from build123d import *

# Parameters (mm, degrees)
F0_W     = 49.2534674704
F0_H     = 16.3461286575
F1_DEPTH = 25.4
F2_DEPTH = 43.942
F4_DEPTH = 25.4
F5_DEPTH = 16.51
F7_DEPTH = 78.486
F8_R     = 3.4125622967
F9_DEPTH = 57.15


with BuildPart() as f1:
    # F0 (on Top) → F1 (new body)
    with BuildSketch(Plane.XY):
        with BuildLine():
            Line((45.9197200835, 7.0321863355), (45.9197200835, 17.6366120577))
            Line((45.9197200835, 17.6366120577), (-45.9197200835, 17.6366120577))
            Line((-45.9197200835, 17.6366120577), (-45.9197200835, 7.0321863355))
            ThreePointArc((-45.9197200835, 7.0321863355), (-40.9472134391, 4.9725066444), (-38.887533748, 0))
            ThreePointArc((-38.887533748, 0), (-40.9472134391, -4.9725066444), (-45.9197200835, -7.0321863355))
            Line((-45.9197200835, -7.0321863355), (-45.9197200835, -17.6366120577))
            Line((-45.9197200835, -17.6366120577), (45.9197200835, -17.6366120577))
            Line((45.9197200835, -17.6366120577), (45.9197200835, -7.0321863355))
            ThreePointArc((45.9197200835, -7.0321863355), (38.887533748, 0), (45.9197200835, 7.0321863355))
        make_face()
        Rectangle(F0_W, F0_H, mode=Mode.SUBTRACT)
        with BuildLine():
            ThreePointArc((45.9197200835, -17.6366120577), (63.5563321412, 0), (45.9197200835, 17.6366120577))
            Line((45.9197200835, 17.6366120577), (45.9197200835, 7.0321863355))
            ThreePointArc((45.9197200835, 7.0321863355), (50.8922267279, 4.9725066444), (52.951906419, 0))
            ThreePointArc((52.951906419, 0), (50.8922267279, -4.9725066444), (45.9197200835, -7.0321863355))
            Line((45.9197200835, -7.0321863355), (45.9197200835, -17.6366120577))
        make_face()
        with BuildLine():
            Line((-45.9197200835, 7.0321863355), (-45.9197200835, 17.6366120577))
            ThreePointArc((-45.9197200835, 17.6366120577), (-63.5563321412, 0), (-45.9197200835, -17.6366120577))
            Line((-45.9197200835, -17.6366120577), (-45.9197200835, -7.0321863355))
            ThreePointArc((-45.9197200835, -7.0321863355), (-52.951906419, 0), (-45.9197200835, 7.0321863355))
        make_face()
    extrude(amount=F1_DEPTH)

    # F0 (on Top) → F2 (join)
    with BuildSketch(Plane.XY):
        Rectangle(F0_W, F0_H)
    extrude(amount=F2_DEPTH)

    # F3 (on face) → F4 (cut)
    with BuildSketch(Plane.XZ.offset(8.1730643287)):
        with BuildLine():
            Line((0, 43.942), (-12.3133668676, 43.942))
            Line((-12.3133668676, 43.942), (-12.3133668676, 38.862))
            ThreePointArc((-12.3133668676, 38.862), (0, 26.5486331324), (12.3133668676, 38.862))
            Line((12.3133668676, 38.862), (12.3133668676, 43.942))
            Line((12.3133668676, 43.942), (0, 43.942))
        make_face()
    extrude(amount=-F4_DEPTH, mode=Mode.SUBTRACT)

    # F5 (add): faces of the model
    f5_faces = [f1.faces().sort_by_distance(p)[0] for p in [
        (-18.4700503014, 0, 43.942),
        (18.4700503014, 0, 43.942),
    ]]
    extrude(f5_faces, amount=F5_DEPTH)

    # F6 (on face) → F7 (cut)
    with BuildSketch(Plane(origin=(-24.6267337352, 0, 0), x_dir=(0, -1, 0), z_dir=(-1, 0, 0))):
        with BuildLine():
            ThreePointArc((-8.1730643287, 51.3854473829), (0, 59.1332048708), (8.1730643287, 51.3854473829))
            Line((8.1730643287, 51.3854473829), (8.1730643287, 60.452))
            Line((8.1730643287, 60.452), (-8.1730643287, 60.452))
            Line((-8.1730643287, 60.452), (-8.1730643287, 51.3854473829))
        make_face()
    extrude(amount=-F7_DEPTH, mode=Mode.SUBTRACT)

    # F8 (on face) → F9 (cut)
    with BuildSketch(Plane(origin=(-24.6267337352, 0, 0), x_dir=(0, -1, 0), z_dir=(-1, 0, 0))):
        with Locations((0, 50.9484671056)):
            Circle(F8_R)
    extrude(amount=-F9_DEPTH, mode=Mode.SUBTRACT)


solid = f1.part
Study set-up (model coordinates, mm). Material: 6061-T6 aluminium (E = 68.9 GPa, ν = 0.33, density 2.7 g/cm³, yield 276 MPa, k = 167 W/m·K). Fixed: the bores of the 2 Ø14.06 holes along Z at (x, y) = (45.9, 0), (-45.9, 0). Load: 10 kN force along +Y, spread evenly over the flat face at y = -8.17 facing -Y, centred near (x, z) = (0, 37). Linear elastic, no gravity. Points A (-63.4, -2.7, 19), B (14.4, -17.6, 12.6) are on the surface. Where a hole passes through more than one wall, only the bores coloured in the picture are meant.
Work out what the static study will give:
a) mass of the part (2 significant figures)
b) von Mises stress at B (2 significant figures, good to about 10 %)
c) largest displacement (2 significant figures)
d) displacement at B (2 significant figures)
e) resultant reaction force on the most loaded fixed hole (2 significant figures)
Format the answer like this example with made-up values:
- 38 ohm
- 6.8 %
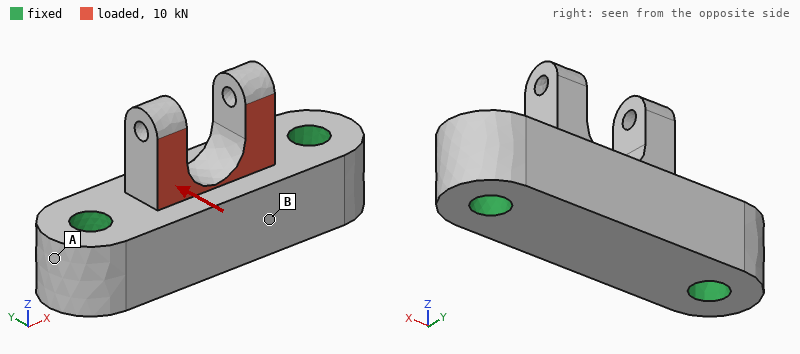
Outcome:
- 300 g
- 20 MPa
- 0.13 mm
- 0.021 mm
- 5.0 kN
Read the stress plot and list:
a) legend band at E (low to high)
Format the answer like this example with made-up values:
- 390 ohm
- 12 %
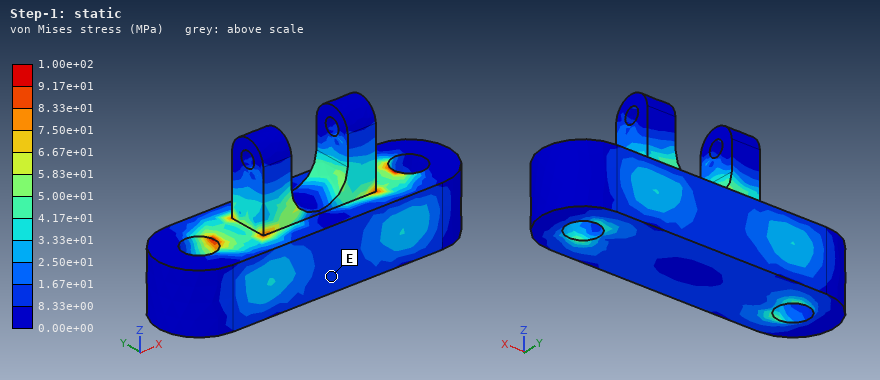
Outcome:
- 8.33e+00 to 1.67e+01 MPa
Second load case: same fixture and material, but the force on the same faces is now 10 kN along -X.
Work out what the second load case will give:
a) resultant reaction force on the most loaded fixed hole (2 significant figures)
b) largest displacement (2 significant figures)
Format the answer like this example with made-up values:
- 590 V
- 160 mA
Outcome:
- 6.0 kN
- 88 µm
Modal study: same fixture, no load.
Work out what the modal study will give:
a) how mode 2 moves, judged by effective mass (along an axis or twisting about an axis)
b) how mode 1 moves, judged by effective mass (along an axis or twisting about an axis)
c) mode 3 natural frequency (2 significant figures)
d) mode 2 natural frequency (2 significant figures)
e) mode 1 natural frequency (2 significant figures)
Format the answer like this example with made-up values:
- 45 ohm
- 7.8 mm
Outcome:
- along Z
- along Y
- 10 kHz
- 9500 Hz
- 7900 Hz
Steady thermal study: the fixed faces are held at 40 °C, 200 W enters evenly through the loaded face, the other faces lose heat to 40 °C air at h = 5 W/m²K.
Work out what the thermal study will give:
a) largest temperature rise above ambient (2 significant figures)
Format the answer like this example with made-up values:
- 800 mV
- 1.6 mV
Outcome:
- 63 K
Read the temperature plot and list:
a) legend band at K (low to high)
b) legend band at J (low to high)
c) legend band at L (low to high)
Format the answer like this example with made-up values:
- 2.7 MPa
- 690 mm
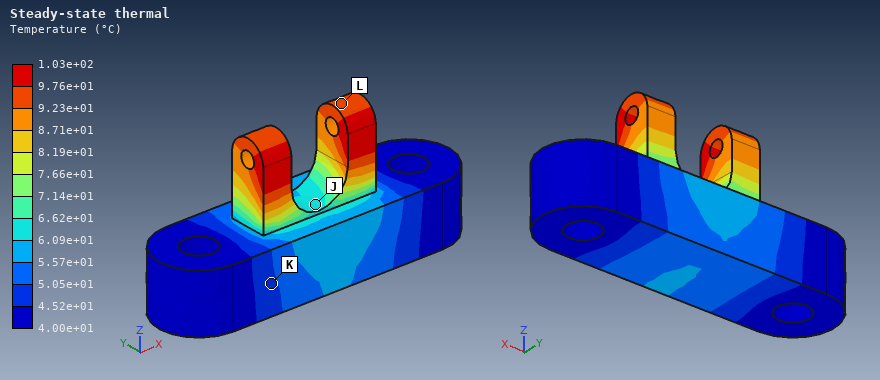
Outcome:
- 4.52e+01 to 5.05e+01 °C
- 6.09e+01 to 6.62e+01 °C
- 9.23e+01 to 9.76e+01 °C
